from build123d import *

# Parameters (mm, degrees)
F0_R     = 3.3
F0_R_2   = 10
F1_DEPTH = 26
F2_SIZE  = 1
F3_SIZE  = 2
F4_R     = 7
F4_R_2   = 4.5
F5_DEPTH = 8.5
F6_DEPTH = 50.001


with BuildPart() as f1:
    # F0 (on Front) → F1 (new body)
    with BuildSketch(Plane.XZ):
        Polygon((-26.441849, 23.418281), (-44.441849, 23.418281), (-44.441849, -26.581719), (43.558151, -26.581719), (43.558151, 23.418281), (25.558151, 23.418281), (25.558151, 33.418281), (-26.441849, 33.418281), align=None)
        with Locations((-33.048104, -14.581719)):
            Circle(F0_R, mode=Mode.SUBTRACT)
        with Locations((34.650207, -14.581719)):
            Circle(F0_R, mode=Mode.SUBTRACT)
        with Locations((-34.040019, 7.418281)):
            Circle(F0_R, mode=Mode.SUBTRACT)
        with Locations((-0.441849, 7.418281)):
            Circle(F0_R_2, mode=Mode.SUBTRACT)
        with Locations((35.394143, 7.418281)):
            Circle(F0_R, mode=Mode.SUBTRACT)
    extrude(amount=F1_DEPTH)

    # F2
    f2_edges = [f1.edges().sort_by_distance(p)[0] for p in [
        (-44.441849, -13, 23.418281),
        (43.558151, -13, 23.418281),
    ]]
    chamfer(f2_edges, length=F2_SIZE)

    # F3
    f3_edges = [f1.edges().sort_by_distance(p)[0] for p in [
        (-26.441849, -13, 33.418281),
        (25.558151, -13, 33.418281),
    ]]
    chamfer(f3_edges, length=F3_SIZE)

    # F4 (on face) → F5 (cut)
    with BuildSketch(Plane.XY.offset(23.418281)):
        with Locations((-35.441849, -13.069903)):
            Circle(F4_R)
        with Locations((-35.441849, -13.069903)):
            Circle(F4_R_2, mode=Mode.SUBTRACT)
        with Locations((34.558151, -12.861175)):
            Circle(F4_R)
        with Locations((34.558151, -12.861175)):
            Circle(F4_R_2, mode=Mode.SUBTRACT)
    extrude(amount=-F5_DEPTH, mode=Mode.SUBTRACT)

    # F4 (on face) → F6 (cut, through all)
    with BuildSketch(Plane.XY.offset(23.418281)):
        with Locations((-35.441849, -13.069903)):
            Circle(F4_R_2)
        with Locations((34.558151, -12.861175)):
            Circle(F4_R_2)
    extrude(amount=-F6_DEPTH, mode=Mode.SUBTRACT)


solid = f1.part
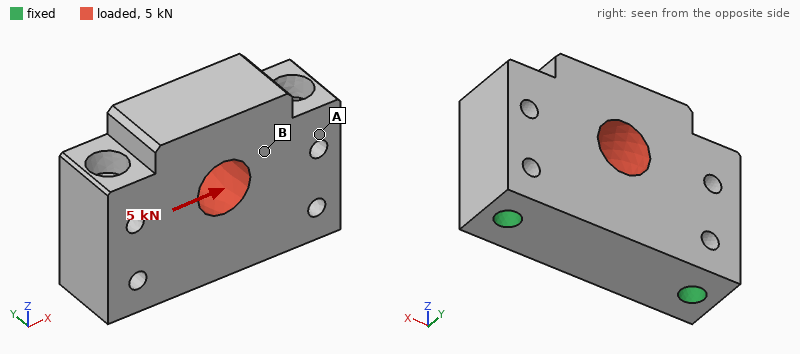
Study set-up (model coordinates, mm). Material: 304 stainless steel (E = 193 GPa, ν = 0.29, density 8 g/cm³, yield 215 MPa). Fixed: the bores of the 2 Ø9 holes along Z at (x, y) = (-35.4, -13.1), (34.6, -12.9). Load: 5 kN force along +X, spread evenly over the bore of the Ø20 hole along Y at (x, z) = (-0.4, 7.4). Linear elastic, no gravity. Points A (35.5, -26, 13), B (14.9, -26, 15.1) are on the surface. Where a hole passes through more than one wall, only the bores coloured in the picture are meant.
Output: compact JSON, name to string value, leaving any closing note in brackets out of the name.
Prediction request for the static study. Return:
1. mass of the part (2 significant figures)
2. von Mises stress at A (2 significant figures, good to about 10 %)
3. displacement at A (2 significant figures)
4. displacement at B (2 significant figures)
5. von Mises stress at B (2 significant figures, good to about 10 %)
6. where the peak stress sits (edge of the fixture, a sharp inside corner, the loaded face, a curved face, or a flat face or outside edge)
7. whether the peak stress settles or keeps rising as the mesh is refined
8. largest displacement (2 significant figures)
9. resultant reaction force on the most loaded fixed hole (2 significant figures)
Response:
{"mass of the part": "870 g", "von Mises stress at A": "1.3 MPa", "displacement at A": "0.25 µm", "displacement at B": "0.50 µm", "von Mises stress at B": "3.7 MPa", "where the peak stress sits": "edge of the fixture", "whether the peak stress settles or keeps rising as the mesh is refined": "keeps rising", "largest displacement": "0.73 µm", "resultant reaction force on the most loaded fixed hole": "2.6 kN"}
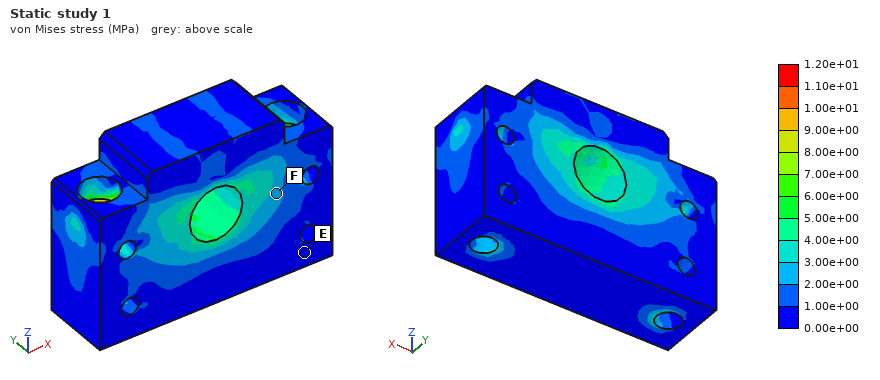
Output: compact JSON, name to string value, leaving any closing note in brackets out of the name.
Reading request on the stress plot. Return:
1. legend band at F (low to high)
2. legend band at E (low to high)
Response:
{"legend band at F": "2.00e+00 to 3.00e+00 MPa", "legend band at E": "0.00e+00 to 1.00e+00 MPa"}
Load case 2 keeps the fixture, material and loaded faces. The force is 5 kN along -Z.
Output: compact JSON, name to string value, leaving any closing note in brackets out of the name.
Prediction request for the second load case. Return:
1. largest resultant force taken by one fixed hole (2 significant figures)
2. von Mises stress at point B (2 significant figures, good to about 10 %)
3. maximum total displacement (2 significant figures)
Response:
{"largest resultant force taken by one fixed hole": "2.6 kN", "von Mises stress at point B": "3.2 MPa", "maximum total displacement": "1.2 µm"}
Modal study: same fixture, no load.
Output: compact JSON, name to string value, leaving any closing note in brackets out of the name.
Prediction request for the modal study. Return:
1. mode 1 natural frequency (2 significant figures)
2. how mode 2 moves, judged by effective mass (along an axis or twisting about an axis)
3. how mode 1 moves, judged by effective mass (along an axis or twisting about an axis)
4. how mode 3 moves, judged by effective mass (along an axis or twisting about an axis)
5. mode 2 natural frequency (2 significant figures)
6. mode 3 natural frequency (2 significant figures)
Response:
{"mode 1 natural frequency": "10 kHz", "how mode 2 moves, judged by effective mass": "along Y", "how mode 1 moves, judged by effective mass": "along Y", "how mode 3 moves, judged by effective mass": "along Z", "mode 2 natural frequency": "15 kHz", "mode 3 natural frequency": "18 kHz"}
